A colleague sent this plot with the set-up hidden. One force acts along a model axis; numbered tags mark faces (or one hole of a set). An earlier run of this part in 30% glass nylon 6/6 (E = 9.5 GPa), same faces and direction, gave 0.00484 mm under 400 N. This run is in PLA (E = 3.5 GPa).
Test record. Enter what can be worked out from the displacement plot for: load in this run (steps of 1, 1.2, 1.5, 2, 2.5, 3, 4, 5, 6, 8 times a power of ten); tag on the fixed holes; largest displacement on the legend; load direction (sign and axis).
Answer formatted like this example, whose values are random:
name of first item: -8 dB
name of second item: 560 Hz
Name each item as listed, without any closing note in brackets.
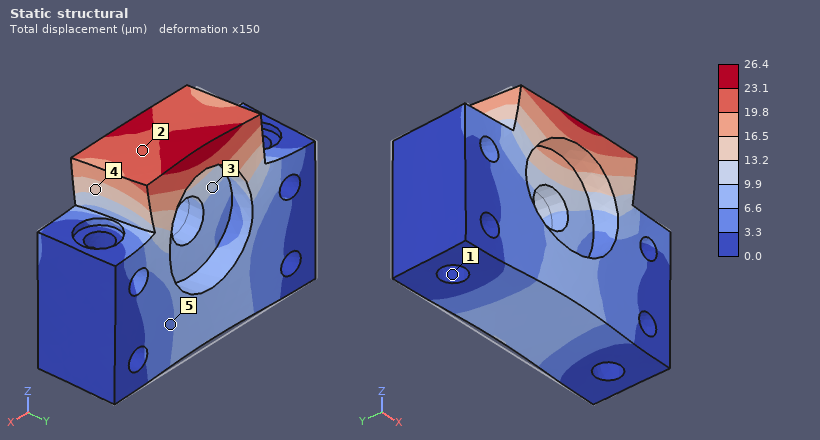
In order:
load in this run: 800 N
tag on the fixed holes: 1
largest displacement on the legend: 26.4 µm
load direction: -Y
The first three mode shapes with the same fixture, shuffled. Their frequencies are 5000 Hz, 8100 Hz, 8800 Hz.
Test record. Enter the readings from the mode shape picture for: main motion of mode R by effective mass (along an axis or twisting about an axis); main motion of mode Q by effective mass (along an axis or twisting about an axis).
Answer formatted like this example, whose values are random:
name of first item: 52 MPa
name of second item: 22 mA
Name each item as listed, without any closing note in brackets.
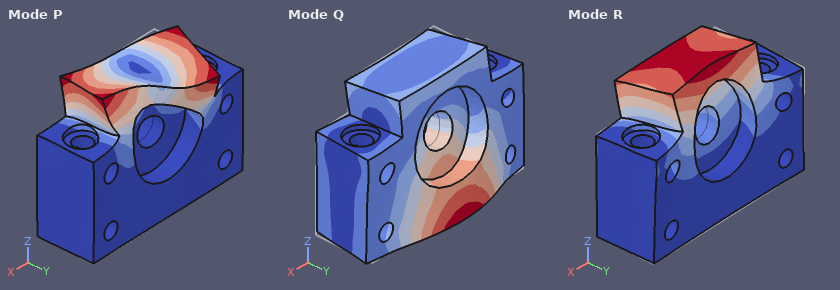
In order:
main motion of mode R by effective mass: along Y
main motion of mode Q by effective mass: along Y
